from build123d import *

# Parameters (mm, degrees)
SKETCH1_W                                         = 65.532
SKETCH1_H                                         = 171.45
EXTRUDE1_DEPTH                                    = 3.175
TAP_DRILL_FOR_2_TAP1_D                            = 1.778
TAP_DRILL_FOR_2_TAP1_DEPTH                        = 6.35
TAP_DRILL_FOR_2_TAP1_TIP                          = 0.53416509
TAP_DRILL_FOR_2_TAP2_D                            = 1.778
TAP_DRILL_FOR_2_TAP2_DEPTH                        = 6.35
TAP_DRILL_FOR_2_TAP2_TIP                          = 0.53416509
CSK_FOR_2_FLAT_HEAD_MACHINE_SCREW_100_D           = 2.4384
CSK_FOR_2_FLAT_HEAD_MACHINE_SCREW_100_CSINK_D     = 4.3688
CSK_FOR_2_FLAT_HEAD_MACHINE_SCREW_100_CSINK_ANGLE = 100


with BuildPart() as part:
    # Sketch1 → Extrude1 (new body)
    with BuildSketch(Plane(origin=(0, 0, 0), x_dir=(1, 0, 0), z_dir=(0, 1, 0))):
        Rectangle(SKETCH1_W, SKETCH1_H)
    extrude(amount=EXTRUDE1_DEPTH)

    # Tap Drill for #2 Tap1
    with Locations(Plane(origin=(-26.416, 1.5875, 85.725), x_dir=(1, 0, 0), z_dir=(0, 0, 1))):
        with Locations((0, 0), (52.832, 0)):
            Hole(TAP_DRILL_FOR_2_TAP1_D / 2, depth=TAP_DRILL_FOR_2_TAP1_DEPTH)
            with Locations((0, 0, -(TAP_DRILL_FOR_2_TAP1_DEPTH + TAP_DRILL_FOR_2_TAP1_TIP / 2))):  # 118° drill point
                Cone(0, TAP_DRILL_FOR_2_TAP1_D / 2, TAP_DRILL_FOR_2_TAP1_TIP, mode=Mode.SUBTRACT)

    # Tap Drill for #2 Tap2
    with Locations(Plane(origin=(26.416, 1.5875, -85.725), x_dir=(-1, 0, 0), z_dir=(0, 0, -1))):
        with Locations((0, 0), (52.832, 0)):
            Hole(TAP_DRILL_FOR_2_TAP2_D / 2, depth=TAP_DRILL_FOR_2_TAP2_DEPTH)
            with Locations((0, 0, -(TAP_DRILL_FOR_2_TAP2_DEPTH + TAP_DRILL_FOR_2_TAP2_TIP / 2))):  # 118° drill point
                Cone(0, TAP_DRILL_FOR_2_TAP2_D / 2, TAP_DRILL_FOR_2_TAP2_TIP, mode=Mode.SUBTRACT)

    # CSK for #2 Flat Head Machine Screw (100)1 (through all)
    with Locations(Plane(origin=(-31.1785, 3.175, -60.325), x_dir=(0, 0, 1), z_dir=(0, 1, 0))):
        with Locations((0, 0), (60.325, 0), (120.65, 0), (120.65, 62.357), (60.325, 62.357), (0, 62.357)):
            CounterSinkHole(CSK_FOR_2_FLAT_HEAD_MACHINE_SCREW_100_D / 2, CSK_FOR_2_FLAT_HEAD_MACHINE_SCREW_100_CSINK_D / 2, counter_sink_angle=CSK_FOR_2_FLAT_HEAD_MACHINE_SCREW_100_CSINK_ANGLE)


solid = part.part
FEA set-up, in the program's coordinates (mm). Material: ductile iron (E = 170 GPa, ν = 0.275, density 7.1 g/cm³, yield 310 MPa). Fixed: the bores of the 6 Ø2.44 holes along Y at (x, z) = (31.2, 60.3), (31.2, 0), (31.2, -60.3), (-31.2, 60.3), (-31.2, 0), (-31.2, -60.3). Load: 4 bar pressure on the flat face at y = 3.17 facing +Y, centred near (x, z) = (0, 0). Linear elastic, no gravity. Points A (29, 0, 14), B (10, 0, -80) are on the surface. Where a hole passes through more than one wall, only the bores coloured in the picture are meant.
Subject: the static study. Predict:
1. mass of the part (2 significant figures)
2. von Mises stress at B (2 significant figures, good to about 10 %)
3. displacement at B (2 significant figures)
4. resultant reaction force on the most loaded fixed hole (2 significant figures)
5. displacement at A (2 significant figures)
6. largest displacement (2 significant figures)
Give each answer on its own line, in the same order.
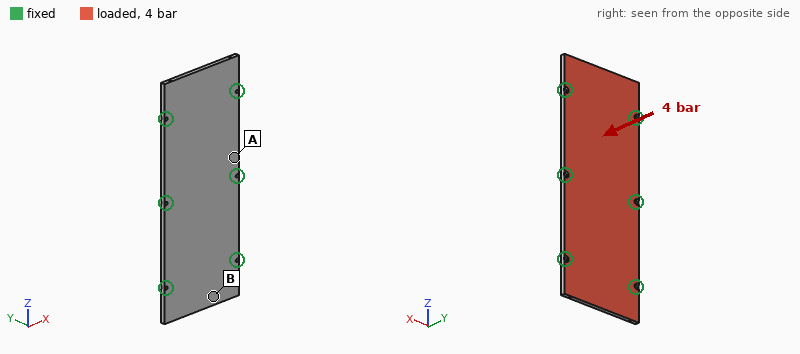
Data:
250 g
52 MPa
0.12 mm
820 N
0.028 mm
0.15 mm
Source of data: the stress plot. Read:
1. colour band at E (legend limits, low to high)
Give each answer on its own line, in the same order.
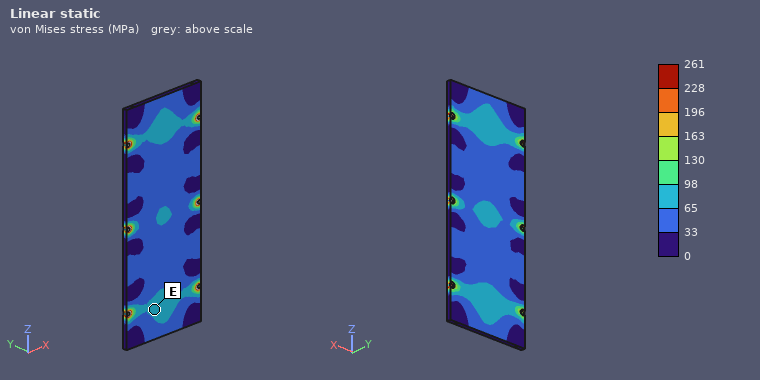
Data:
65 to 98 MPa
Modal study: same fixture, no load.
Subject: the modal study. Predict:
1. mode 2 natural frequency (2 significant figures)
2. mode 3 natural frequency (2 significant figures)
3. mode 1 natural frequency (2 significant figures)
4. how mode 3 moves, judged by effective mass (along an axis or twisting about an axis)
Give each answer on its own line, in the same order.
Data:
2100 Hz
2400 Hz
2100 Hz
along Y
